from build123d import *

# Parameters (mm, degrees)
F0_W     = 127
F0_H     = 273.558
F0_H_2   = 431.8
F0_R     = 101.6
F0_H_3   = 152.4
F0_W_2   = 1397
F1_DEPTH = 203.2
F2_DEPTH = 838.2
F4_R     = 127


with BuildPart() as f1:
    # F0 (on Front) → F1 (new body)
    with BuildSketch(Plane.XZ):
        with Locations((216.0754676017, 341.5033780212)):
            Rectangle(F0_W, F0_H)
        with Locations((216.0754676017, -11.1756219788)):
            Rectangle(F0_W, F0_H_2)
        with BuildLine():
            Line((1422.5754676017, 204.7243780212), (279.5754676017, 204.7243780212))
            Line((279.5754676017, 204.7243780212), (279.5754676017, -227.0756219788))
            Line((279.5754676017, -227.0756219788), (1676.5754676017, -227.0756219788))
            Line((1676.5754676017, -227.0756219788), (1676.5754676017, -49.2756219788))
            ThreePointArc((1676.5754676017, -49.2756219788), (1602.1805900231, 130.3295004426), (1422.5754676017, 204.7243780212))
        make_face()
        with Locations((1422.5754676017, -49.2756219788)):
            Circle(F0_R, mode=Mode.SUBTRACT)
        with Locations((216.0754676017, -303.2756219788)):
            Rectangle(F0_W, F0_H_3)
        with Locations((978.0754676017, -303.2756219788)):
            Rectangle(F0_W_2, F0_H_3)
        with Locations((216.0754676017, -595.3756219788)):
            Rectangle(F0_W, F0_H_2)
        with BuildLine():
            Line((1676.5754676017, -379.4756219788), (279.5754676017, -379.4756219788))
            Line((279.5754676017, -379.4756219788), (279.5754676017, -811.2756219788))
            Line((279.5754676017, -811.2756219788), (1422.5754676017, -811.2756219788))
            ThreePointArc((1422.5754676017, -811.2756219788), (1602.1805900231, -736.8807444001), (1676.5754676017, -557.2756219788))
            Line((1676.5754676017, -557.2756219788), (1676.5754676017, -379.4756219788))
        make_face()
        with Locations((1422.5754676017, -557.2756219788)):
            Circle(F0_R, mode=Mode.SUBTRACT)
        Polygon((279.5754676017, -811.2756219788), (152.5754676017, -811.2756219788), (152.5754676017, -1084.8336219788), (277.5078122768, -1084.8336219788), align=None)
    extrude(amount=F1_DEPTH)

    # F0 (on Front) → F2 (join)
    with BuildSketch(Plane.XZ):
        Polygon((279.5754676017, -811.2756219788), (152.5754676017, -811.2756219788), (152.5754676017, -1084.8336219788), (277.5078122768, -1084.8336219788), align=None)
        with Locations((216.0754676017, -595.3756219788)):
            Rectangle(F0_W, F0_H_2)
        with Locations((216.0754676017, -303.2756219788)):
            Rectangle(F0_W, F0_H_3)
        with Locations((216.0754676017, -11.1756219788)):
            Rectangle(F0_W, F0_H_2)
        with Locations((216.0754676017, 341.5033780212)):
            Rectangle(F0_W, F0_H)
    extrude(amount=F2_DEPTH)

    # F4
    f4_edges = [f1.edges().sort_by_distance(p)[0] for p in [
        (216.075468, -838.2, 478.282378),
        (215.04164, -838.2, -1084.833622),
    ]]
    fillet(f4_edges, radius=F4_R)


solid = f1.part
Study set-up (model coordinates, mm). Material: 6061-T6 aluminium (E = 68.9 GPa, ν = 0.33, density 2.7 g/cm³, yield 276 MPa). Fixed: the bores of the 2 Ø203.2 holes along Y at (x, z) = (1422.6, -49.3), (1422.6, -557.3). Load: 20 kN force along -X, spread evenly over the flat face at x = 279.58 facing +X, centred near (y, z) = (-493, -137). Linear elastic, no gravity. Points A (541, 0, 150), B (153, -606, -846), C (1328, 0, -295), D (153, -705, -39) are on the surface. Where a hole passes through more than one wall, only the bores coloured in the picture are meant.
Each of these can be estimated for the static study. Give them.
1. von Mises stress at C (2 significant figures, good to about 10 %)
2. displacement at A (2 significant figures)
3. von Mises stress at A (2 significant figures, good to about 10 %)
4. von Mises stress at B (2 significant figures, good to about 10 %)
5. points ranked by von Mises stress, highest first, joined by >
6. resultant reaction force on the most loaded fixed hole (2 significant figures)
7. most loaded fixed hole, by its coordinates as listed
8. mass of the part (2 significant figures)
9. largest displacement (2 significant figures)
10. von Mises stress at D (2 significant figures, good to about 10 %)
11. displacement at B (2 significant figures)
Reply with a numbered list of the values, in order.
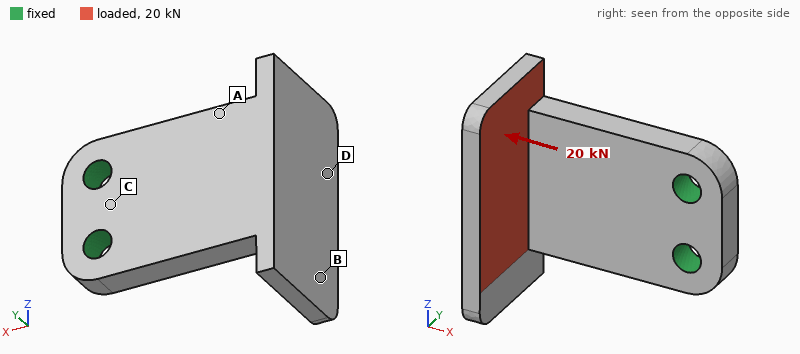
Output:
1. 0.63 MPa
2. 0.053 mm
3. 1.1 MPa
4. 0.31 MPa
5. A > C > B > D
6. 15 kN
7. (1422.6, -49.3)
8. 1200 kg
9. 0.23 mm
10. 0.16 MPa
11. 0.16 mm
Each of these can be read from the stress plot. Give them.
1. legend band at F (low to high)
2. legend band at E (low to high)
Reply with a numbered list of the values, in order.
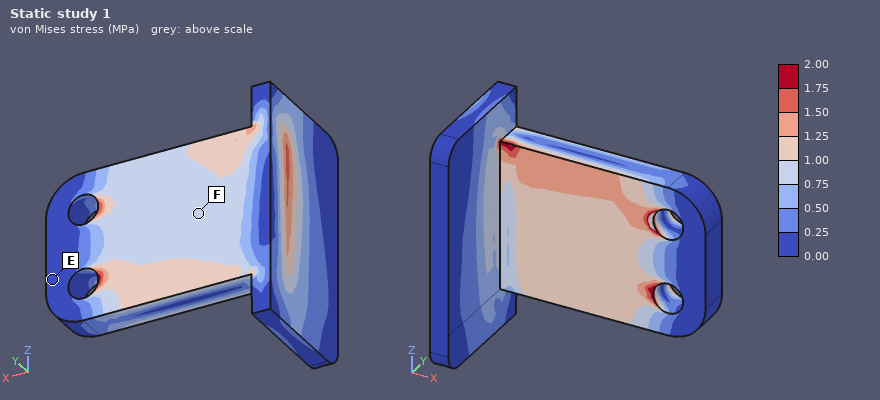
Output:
1. 0.75 to 1.00 MPa
2. 0.00 to 0.25 MPa
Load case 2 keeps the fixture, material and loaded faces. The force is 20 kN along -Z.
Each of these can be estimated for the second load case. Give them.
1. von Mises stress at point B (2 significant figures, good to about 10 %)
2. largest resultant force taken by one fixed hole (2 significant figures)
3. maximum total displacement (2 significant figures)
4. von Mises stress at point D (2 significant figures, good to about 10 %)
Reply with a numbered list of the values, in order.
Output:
1. 0.16 MPa
2. 37 kN
3. 0.12 mm
4. 0.19 MPa
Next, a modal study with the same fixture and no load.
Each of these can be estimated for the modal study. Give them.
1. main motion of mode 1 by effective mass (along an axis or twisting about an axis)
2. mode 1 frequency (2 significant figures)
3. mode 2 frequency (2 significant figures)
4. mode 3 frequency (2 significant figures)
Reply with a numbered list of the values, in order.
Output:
1. along Y
2. 59 Hz
3. 100 Hz
4. 170 Hz
